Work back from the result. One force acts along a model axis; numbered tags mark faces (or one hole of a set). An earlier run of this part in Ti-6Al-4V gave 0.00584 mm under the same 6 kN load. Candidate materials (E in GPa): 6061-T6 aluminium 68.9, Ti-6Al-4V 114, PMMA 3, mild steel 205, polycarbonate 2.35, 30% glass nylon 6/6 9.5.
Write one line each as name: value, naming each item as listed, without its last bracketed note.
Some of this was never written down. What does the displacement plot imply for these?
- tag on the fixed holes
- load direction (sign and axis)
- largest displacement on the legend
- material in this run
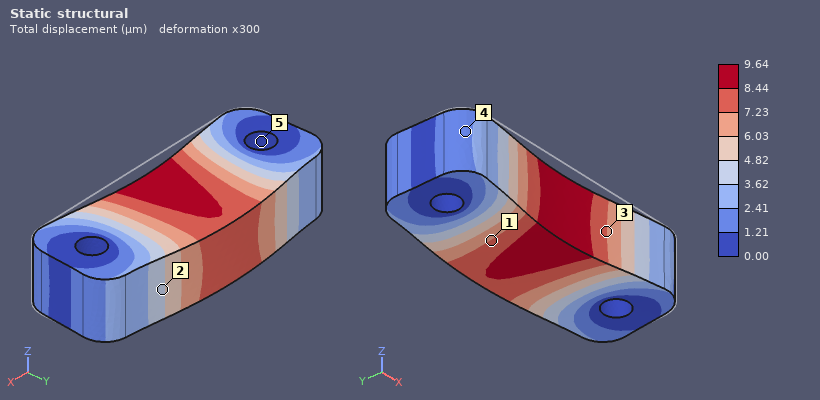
tag on the fixed holes: 5
load direction: +Y
largest displacement on the legend: 9.64 µm
material in this run: 6061-T6 aluminium
